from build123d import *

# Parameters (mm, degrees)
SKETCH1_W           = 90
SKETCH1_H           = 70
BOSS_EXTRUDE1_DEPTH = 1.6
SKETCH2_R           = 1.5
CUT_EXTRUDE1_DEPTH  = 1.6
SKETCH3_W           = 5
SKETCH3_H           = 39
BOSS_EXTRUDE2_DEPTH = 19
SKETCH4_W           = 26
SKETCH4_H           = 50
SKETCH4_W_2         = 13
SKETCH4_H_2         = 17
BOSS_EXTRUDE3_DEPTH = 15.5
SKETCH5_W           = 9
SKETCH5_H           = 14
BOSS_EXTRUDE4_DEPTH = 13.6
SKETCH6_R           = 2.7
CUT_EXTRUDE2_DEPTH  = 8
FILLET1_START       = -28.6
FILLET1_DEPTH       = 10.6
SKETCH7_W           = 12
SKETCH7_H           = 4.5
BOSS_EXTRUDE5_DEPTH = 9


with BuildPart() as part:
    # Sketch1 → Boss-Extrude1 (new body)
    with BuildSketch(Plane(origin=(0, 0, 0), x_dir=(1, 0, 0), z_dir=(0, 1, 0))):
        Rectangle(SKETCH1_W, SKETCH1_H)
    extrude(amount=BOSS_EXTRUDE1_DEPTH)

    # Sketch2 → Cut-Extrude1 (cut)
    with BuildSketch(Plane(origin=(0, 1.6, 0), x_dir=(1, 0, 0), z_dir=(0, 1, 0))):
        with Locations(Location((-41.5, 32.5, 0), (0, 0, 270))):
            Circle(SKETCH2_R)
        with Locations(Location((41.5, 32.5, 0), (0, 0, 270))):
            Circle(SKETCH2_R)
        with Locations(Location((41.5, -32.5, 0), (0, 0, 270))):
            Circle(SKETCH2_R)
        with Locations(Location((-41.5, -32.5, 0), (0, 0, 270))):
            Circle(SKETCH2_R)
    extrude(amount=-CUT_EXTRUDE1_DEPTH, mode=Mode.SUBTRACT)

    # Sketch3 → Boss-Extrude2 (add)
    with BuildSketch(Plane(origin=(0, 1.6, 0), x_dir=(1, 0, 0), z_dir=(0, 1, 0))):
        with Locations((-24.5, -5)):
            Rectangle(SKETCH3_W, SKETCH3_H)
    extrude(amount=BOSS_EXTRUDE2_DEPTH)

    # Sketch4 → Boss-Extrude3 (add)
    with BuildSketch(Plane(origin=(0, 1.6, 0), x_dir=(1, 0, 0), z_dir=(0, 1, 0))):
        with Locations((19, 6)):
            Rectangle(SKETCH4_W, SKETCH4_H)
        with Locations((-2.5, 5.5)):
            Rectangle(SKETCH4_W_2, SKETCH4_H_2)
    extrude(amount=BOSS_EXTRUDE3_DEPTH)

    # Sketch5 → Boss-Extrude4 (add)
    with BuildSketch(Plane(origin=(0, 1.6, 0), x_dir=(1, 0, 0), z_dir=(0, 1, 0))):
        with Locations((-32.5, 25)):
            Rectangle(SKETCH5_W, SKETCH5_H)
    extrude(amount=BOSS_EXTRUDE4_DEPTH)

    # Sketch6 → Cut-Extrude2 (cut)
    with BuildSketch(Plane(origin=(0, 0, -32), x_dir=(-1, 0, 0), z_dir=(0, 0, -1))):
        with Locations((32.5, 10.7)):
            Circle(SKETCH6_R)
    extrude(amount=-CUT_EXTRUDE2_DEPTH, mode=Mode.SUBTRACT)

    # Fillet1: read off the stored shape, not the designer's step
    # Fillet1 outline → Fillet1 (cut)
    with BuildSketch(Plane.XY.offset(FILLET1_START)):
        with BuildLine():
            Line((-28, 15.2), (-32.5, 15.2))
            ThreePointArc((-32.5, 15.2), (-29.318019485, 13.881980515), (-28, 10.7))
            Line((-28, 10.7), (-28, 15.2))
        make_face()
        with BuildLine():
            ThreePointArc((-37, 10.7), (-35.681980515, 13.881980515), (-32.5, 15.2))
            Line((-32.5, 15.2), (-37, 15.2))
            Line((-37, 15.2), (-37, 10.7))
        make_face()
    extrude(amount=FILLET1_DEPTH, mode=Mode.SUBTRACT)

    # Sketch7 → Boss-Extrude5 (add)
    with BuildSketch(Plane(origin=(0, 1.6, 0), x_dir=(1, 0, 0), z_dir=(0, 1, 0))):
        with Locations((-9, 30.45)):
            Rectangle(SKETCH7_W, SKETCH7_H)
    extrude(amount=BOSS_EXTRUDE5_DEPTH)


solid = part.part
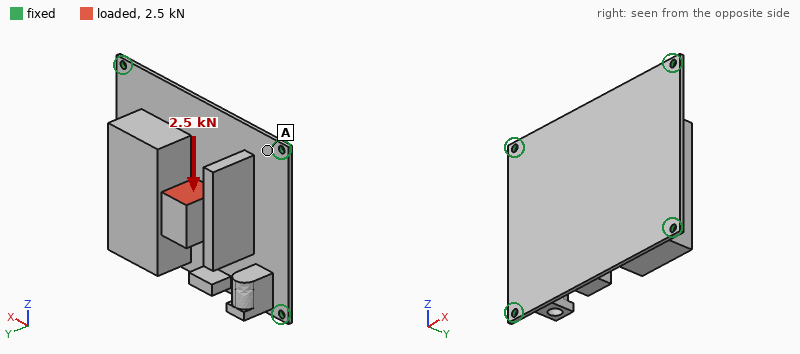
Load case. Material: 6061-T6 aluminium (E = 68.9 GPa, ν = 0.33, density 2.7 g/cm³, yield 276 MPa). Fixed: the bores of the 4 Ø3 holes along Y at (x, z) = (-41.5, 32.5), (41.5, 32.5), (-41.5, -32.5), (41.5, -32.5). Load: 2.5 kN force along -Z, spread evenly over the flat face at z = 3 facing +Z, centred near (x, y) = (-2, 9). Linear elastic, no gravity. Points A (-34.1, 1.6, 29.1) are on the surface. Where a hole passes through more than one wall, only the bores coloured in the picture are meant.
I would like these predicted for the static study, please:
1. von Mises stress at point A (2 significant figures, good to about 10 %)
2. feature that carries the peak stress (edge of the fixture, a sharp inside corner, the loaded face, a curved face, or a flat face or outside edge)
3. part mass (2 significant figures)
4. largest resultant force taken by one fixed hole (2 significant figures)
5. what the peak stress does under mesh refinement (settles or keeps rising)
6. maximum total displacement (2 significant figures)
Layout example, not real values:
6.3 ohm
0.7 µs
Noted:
40 MPa
edge of the fixture
110 g
960 N
keeps rising
0.32 mm
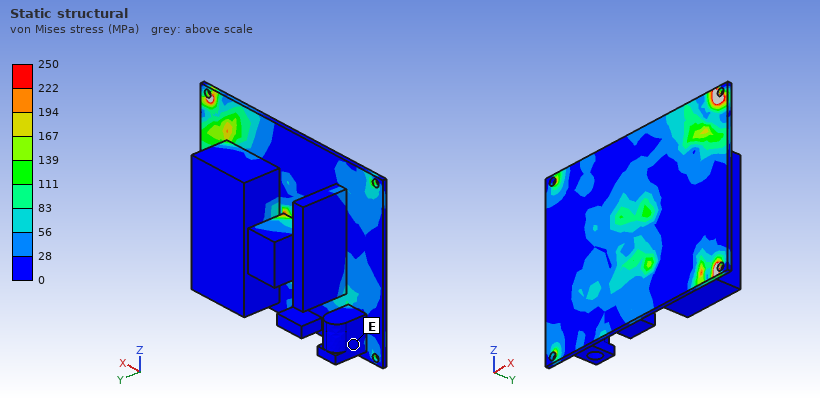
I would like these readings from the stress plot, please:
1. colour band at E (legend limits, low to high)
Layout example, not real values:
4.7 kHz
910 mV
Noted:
0 to 28 MPa
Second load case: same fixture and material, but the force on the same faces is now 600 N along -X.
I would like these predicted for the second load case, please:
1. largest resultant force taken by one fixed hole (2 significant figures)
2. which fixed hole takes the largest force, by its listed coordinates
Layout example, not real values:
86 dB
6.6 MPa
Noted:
220 N
(41.5, -32.5)
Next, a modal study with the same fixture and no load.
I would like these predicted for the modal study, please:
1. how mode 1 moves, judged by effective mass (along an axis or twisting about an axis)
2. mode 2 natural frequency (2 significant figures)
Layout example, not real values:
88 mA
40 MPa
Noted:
along Y
1400 Hz
